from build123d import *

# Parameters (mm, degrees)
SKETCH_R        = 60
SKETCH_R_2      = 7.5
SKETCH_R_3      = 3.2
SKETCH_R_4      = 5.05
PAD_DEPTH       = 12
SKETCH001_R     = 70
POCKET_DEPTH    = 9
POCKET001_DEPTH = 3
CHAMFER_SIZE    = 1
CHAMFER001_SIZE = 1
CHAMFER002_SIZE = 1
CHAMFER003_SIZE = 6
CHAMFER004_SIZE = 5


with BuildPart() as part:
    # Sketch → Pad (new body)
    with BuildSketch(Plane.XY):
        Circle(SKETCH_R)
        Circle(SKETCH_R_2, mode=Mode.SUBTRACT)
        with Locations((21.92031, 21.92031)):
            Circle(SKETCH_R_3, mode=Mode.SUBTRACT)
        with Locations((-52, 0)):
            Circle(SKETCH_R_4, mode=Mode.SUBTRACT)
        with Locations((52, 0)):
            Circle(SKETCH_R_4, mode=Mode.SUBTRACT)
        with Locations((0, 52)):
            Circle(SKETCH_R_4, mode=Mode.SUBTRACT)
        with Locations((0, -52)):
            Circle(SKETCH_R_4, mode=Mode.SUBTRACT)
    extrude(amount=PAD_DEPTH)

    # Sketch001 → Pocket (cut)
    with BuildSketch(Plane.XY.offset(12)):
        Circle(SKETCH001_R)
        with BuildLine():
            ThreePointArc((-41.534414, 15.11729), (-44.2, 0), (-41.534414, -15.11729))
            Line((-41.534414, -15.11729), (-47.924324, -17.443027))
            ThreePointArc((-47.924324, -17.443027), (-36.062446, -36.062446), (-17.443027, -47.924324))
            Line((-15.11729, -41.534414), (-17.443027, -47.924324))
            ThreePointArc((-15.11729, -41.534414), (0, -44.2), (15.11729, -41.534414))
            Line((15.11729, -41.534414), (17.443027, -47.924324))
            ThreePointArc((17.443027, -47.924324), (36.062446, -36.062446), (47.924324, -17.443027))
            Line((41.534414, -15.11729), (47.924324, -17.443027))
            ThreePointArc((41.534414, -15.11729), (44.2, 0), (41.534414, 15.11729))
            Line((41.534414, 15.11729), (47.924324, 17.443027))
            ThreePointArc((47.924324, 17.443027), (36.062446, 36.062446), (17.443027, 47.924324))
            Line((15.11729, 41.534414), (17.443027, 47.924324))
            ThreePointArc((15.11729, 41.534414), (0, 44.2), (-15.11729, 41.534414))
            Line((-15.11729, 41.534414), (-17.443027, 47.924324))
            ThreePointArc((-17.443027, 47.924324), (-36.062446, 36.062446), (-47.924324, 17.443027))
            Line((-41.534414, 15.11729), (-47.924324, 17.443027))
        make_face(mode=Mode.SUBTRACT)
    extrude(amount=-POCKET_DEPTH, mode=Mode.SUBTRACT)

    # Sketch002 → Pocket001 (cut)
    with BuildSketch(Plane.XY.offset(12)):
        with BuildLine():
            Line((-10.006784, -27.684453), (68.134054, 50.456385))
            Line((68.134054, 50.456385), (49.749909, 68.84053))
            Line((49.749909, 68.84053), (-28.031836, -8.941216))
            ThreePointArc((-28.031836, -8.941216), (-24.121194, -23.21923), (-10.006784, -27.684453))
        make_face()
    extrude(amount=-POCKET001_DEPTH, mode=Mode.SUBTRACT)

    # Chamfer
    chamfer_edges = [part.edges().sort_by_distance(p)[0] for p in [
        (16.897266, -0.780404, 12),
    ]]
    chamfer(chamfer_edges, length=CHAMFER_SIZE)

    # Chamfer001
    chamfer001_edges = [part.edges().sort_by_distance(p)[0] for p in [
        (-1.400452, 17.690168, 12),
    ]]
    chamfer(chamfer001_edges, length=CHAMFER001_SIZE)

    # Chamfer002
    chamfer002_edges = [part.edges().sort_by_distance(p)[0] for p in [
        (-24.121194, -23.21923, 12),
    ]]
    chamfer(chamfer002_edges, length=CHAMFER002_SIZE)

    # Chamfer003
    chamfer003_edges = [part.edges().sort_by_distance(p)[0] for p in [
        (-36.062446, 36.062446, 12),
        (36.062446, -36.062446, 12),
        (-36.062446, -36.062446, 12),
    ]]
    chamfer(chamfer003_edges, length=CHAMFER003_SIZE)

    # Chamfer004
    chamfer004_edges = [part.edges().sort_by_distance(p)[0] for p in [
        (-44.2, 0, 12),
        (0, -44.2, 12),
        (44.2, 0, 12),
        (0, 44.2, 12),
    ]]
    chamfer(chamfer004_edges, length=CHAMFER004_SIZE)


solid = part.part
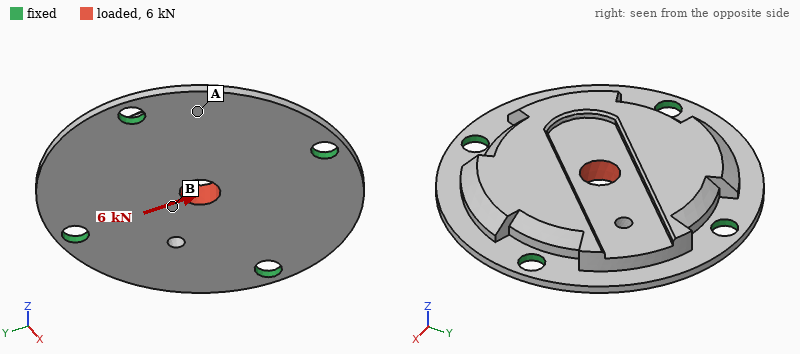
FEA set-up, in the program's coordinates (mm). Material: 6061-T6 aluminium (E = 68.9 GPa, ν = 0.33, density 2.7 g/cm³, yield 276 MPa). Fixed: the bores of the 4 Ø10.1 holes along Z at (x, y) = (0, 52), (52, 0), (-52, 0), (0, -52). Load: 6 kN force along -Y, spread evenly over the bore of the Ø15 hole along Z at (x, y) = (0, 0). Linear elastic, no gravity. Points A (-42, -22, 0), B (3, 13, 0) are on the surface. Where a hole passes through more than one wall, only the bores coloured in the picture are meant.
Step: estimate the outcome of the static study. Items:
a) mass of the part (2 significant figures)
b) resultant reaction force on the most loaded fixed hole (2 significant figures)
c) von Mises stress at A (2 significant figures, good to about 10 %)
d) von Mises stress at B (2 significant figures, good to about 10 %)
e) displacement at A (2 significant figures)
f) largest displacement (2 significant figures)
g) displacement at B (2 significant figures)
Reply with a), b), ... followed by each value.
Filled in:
a) 230 g
b) 1.9 kN
c) 5.2 MPa
d) 13 MPa
e) 3.6 µm
f) 9.5 µm
g) 8.3 µm
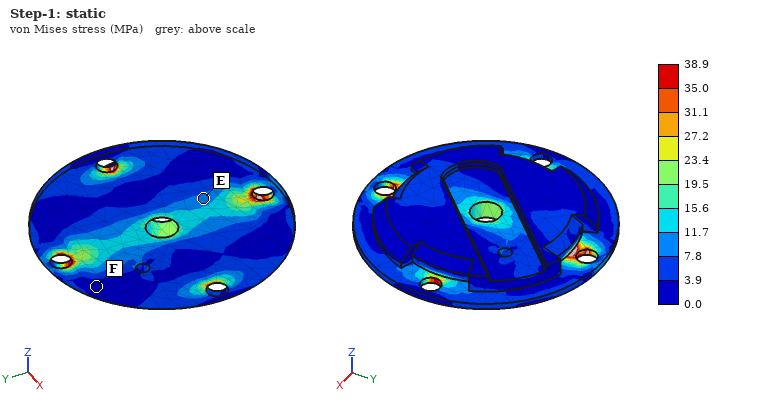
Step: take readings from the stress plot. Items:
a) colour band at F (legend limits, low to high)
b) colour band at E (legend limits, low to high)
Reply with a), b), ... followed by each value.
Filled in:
a) 0.0 to 3.9 MPa
b) 7.8 to 11.7 MPa
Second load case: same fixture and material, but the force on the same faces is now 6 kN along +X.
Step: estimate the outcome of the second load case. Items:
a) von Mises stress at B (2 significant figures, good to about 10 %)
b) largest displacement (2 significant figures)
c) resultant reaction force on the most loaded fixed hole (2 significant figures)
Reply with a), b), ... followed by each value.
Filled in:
a) 6.1 MPa
b) 9.5 µm
c) 1.9 kN
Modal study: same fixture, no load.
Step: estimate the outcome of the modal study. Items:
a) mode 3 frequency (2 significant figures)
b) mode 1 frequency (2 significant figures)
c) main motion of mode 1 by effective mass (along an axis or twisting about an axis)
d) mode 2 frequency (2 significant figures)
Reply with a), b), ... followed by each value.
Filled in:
a) 5900 Hz
b) 4700 Hz
c) along Z
d) 5600 Hz
